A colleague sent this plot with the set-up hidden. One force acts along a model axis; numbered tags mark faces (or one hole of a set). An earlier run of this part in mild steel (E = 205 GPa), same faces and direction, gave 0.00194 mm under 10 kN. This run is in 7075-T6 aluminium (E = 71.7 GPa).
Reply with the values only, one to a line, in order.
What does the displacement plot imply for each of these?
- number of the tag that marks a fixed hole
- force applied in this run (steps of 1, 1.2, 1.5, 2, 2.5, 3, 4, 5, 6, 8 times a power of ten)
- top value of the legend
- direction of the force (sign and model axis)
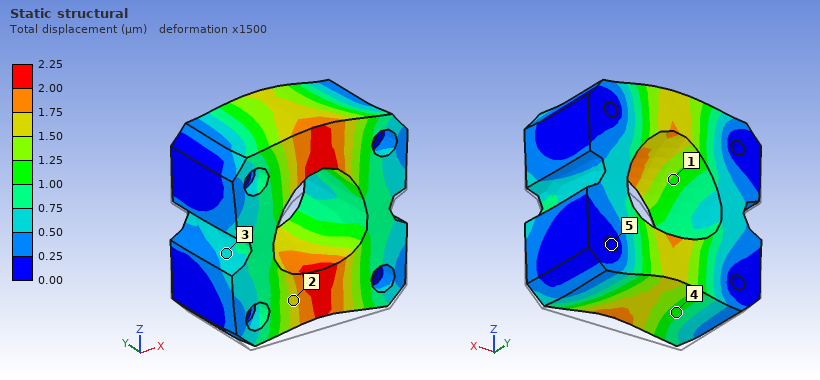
5
4 kN
2.25 µm
+Z
